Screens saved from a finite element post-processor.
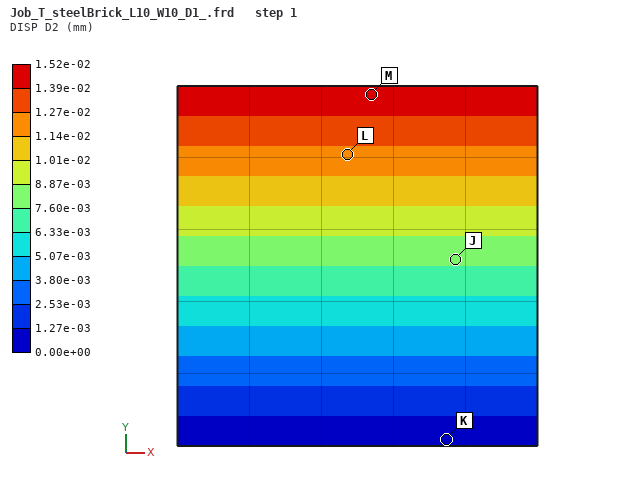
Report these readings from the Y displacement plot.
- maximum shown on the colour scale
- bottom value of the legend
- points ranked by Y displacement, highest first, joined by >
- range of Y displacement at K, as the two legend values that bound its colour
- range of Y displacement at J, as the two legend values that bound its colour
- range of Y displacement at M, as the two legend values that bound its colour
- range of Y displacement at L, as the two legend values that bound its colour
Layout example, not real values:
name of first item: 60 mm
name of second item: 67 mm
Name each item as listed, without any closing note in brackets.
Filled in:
maximum shown on the colour scale: 1.52e-02 mm
bottom value of the legend: 0.00e+00 mm
points ranked by Y displacement, highest first, joined by >: M > L > J > K
range of Y displacement at K, as the two legend values that bound its colour: 0.00e+00 to 1.27e-03 mm
range of Y displacement at J, as the two legend values that bound its colour: 7.60e-03 to 8.87e-03 mm
range of Y displacement at M, as the two legend values that bound its colour: 1.39e-02 to 1.52e-02 mm
range of Y displacement at L, as the two legend values that bound its colour: 1.14e-02 to 1.27e-02 mm
